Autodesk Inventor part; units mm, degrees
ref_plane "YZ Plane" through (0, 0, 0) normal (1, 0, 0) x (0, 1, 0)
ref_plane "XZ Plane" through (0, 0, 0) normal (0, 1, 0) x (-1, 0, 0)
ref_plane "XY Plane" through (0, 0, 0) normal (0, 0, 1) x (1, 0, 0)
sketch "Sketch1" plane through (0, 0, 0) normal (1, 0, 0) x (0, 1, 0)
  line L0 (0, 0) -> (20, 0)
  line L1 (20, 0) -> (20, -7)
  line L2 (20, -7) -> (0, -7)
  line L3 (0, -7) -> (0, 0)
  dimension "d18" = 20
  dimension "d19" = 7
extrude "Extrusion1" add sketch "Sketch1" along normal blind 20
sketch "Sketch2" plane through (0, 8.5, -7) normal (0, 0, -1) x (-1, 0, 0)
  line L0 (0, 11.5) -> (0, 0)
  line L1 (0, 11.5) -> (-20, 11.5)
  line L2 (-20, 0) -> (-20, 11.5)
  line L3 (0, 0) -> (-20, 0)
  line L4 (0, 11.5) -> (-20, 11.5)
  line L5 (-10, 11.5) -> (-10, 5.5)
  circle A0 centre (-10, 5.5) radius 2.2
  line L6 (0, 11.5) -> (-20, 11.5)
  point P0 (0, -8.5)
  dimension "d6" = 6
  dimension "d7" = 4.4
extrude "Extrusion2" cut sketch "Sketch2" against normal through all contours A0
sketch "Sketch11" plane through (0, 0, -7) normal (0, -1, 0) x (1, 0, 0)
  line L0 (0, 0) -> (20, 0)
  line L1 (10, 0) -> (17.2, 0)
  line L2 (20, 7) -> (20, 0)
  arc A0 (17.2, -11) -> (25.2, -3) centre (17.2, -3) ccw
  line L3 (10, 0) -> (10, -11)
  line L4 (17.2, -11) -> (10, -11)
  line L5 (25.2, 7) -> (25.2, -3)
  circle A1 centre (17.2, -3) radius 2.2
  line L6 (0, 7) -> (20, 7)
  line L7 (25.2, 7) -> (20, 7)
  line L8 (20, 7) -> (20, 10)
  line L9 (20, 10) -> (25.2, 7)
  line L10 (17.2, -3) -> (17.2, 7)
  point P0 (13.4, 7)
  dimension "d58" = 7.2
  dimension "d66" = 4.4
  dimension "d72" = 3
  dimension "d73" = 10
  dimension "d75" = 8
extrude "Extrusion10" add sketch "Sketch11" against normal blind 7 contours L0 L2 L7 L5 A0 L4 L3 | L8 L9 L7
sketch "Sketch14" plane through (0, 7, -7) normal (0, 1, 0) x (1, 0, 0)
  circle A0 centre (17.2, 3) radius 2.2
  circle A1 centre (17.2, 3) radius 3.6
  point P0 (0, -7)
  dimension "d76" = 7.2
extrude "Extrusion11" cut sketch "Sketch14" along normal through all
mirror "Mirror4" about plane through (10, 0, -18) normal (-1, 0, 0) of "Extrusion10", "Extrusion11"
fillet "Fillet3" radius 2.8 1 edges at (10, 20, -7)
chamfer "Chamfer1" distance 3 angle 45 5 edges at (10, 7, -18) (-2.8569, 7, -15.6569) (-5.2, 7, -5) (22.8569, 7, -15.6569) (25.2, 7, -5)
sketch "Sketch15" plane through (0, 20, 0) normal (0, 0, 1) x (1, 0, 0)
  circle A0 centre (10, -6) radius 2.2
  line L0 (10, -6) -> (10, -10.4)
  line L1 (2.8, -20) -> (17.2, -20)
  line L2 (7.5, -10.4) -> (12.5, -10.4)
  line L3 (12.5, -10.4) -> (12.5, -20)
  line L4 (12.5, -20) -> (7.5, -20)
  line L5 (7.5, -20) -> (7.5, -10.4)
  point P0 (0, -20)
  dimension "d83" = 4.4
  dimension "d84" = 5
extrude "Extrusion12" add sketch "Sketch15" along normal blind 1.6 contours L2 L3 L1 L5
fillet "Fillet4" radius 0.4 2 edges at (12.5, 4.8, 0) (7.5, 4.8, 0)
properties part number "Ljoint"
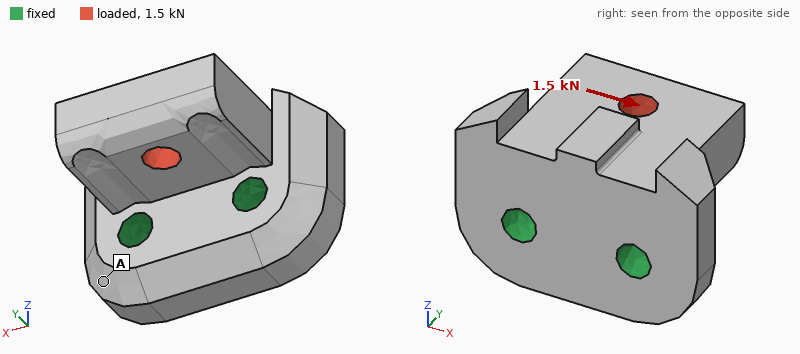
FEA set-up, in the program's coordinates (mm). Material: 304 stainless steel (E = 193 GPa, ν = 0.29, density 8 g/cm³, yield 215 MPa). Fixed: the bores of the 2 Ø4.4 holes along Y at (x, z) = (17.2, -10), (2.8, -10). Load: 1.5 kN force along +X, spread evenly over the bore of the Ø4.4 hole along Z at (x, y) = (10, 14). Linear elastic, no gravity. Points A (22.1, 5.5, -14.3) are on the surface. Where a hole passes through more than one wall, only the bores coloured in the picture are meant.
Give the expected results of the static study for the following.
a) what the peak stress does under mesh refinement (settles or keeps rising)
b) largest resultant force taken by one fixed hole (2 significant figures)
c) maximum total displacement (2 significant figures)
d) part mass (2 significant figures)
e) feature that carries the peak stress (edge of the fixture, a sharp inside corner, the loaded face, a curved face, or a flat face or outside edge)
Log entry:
keeps rising
1.2 kN
5.6 µm
40 g
edge of the fixture
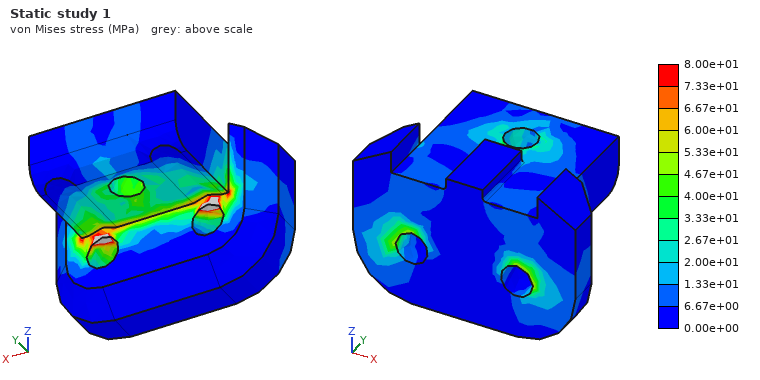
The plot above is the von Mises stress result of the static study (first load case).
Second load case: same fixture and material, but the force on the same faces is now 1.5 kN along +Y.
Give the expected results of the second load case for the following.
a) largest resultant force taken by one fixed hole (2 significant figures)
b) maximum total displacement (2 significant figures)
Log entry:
760 N
5.1 µm
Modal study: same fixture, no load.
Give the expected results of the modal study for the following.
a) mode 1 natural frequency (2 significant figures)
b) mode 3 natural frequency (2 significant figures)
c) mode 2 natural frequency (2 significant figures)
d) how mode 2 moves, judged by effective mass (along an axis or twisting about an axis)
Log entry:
15 kHz
32 kHz
25 kHz
along X
